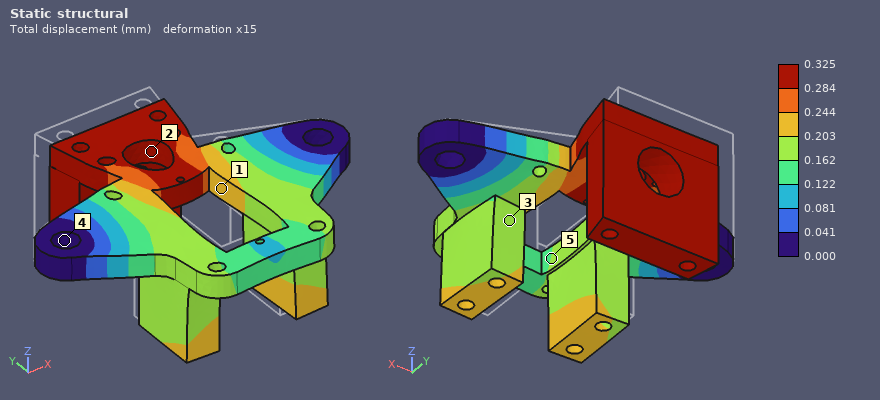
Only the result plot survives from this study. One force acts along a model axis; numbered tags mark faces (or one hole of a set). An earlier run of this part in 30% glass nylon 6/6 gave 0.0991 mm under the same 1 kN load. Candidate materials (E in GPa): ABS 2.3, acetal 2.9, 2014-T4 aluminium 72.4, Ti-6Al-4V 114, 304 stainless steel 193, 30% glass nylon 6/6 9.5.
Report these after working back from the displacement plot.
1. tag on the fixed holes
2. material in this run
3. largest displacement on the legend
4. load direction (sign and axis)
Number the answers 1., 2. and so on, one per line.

1. 4
2. acetal
3. 0.325 mm
4. -Y
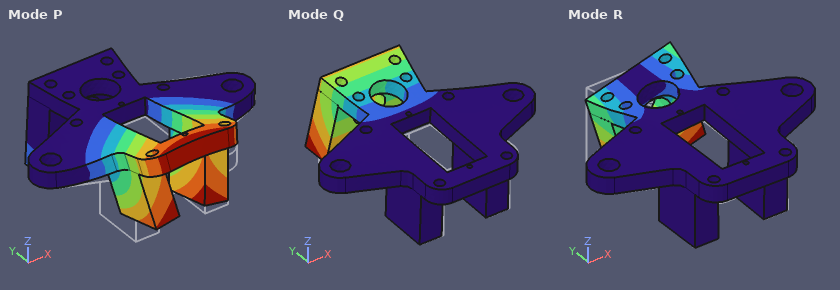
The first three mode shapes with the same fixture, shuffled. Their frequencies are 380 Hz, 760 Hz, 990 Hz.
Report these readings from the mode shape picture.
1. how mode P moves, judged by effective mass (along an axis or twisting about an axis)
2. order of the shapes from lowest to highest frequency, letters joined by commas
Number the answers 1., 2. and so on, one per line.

1. along Z
2. Q, R, P
